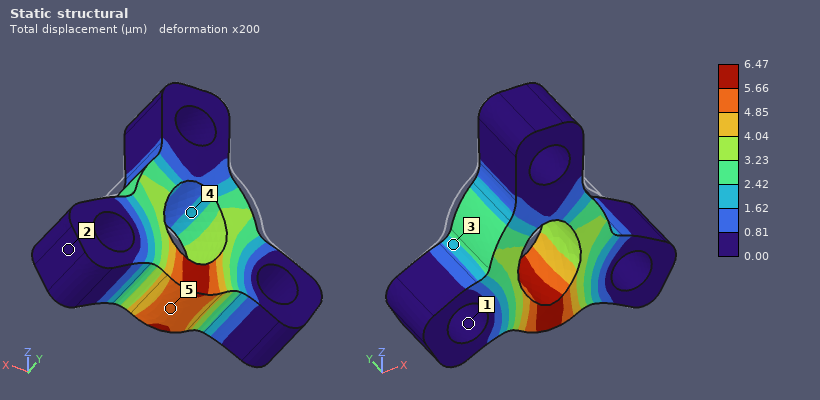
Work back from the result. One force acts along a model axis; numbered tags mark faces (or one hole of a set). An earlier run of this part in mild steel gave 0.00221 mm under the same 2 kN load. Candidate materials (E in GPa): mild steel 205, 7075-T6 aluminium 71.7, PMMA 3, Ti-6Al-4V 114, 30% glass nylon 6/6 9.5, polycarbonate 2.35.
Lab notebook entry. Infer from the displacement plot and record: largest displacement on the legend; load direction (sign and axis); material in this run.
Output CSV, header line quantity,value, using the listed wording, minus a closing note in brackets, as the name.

quantity,value
largest displacement on the legend,6.47 µm
load direction,-Z
material in this run,7075-T6 aluminium
